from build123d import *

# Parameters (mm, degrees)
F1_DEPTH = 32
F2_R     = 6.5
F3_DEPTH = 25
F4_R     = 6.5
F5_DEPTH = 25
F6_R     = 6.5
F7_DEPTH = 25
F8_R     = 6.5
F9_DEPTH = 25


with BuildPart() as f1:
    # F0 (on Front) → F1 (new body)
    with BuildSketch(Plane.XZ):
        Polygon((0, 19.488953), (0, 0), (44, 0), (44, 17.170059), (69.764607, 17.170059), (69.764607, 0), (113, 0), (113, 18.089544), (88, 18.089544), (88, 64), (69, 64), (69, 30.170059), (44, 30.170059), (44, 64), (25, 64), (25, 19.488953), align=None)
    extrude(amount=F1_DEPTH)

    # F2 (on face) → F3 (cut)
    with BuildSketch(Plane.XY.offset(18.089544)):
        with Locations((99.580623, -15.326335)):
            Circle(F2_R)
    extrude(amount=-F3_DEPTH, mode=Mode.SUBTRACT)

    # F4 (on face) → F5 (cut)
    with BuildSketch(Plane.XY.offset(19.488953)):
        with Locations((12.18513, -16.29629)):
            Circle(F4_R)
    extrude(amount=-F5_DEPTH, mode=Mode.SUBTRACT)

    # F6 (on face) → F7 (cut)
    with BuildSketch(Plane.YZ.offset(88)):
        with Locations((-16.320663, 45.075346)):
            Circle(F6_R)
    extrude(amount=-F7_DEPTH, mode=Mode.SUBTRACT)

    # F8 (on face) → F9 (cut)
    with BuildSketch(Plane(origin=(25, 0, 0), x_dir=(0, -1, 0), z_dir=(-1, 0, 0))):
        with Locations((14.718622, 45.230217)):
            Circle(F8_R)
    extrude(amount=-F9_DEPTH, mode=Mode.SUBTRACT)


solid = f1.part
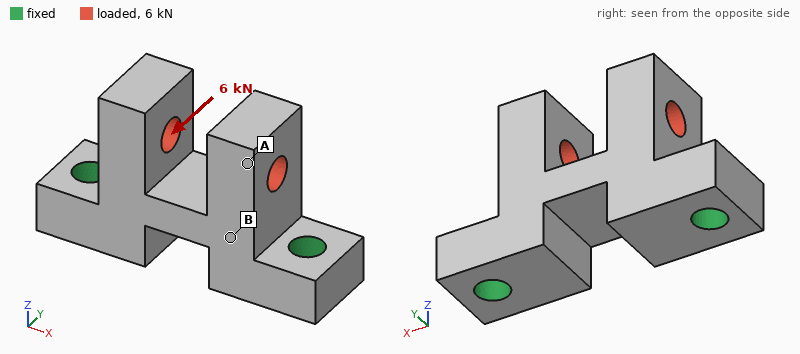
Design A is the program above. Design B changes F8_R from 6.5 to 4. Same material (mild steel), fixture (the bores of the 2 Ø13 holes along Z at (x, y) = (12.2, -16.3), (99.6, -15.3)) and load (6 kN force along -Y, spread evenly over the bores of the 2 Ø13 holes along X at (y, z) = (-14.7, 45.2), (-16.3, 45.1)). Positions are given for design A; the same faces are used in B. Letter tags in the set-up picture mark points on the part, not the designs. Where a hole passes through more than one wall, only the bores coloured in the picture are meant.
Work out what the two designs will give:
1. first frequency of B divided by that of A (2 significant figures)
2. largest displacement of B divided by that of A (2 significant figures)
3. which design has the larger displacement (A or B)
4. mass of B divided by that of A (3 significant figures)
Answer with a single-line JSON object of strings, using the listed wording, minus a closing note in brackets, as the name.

{"first frequency of B divided by that of A": "0.99", "largest displacement of B divided by that of A": "1.1", "which design has the larger displacement": "B", "mass of B divided by that of A": "1.01"}
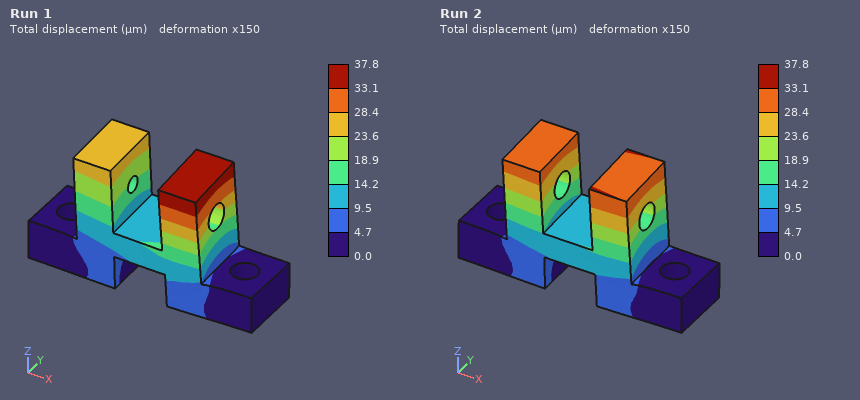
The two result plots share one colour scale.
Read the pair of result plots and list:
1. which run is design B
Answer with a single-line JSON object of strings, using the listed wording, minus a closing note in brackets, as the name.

{"which run is design B": "Run 1"}
